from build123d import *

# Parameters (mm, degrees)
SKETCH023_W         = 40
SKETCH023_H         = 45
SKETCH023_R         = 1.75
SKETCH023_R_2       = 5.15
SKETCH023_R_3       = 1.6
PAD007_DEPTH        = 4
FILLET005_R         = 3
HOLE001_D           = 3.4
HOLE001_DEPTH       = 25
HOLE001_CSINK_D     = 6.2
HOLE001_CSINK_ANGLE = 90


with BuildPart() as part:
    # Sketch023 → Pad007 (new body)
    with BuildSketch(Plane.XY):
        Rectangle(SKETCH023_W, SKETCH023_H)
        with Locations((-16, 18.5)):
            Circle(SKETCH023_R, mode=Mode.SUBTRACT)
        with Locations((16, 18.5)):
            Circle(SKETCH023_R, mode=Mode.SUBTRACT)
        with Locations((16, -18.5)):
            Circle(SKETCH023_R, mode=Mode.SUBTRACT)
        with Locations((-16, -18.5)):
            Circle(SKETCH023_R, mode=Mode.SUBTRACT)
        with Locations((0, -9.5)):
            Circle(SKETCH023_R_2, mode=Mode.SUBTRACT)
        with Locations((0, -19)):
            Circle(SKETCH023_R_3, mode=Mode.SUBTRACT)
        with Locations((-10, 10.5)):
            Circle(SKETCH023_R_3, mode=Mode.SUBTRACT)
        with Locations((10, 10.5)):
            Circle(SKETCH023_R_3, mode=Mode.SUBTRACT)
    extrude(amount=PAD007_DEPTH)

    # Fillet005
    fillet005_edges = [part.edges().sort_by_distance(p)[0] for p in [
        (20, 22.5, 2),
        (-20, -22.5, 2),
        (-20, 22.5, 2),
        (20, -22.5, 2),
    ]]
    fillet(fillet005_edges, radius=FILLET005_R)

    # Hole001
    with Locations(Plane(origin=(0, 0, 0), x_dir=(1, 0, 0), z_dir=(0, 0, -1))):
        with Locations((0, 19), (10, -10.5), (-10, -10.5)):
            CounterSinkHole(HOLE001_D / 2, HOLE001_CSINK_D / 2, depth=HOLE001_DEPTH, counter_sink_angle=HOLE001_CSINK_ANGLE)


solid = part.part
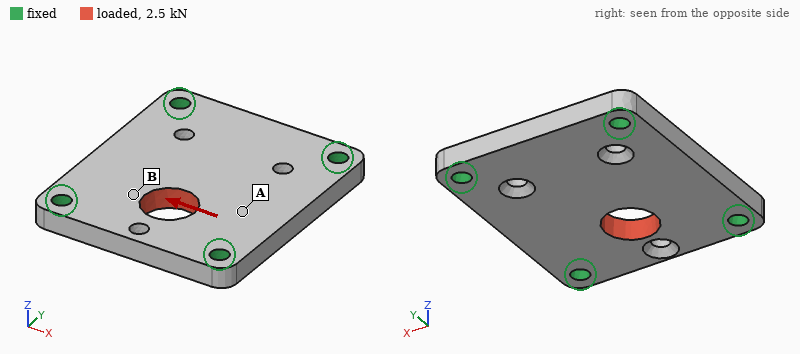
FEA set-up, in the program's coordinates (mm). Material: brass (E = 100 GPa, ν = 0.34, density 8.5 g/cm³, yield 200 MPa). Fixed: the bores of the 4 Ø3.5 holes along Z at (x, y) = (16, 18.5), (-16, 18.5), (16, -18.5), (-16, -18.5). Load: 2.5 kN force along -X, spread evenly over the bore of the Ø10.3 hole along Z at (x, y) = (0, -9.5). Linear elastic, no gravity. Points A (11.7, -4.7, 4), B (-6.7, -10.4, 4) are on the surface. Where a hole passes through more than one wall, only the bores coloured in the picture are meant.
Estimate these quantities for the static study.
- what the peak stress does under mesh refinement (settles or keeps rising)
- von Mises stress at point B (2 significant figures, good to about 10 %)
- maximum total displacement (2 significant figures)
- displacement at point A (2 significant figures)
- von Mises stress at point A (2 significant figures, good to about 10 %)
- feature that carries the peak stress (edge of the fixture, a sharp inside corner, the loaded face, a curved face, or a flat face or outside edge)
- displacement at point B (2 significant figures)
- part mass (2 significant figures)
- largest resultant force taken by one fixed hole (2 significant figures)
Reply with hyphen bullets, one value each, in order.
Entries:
- keeps rising
- 21 MPa
- 5.2 µm
- 4.0 µm
- 7.6 MPa
- edge of the fixture
- 4.0 µm
- 56 g
- 920 N
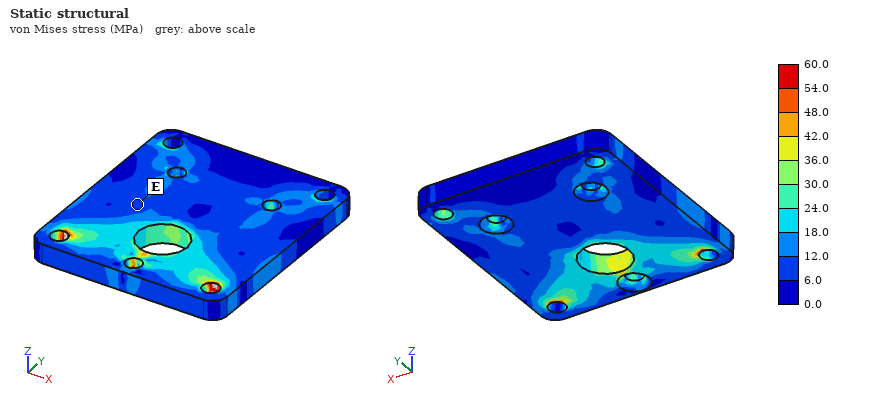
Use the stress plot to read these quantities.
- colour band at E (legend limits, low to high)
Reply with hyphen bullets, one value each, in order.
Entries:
- 6.0 to 12.0 MPa
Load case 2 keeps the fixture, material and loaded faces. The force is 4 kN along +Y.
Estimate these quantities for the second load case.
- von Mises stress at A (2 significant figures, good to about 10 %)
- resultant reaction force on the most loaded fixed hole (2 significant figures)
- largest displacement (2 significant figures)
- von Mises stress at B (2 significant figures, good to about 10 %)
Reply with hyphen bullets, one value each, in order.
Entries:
- 24 MPa
- 1.3 kN
- 12 µm
- 48 MPa
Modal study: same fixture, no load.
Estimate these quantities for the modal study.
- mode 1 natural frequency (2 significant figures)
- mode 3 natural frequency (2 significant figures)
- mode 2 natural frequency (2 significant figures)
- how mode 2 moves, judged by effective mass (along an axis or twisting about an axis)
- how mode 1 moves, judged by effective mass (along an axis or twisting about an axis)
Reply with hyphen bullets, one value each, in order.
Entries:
- 7700 Hz
- 14 kHz
- 11 kHz
- twisting about Y
- along Z
